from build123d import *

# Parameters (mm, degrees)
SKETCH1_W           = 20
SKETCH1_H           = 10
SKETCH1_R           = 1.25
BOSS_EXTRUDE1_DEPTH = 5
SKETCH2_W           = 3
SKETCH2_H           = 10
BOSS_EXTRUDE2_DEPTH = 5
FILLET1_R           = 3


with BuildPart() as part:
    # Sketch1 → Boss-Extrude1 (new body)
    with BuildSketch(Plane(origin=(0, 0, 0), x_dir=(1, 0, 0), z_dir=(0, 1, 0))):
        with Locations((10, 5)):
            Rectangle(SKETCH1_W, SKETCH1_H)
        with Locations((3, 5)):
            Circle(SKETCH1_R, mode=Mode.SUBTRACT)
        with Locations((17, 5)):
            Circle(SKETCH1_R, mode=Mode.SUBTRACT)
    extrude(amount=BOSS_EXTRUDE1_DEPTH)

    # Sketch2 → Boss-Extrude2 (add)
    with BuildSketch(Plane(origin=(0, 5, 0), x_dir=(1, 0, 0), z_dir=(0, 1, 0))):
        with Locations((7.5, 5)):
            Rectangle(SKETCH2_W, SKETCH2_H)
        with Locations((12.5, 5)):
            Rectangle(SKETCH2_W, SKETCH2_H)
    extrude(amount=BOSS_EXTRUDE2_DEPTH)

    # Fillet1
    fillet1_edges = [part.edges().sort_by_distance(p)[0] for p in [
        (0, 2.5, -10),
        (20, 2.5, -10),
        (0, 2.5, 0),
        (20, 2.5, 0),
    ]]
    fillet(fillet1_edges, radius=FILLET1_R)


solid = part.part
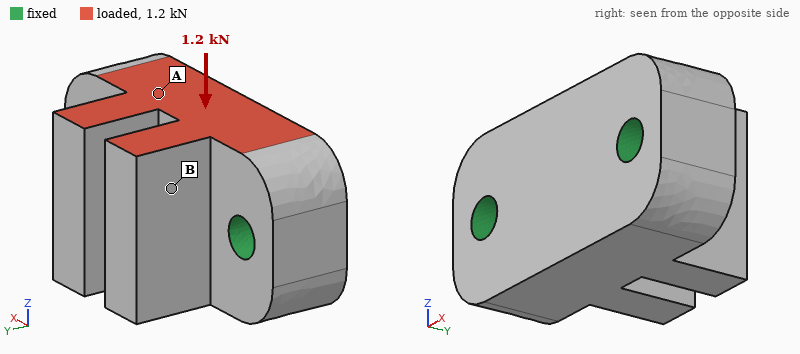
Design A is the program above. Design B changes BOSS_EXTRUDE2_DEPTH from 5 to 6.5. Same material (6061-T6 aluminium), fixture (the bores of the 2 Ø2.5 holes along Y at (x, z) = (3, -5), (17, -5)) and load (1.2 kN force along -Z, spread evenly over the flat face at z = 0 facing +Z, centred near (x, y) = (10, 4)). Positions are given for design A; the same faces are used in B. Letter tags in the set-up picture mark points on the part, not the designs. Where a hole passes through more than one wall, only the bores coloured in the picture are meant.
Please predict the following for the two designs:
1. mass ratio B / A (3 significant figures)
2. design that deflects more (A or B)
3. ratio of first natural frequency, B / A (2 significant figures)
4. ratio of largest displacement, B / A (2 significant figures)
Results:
1.07
B
0.82
1.4
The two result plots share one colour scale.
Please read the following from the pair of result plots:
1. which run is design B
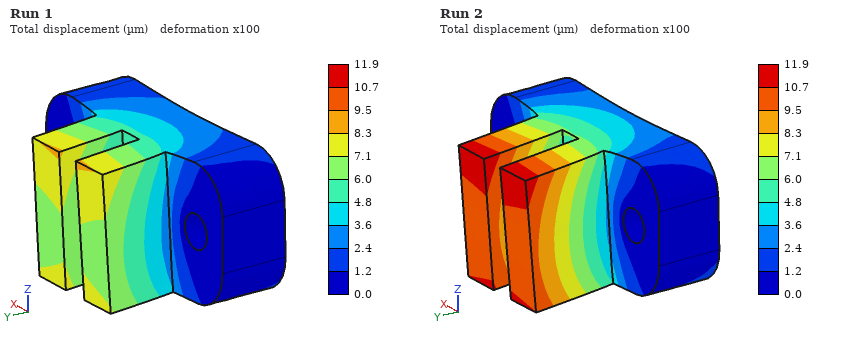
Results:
Run 2
